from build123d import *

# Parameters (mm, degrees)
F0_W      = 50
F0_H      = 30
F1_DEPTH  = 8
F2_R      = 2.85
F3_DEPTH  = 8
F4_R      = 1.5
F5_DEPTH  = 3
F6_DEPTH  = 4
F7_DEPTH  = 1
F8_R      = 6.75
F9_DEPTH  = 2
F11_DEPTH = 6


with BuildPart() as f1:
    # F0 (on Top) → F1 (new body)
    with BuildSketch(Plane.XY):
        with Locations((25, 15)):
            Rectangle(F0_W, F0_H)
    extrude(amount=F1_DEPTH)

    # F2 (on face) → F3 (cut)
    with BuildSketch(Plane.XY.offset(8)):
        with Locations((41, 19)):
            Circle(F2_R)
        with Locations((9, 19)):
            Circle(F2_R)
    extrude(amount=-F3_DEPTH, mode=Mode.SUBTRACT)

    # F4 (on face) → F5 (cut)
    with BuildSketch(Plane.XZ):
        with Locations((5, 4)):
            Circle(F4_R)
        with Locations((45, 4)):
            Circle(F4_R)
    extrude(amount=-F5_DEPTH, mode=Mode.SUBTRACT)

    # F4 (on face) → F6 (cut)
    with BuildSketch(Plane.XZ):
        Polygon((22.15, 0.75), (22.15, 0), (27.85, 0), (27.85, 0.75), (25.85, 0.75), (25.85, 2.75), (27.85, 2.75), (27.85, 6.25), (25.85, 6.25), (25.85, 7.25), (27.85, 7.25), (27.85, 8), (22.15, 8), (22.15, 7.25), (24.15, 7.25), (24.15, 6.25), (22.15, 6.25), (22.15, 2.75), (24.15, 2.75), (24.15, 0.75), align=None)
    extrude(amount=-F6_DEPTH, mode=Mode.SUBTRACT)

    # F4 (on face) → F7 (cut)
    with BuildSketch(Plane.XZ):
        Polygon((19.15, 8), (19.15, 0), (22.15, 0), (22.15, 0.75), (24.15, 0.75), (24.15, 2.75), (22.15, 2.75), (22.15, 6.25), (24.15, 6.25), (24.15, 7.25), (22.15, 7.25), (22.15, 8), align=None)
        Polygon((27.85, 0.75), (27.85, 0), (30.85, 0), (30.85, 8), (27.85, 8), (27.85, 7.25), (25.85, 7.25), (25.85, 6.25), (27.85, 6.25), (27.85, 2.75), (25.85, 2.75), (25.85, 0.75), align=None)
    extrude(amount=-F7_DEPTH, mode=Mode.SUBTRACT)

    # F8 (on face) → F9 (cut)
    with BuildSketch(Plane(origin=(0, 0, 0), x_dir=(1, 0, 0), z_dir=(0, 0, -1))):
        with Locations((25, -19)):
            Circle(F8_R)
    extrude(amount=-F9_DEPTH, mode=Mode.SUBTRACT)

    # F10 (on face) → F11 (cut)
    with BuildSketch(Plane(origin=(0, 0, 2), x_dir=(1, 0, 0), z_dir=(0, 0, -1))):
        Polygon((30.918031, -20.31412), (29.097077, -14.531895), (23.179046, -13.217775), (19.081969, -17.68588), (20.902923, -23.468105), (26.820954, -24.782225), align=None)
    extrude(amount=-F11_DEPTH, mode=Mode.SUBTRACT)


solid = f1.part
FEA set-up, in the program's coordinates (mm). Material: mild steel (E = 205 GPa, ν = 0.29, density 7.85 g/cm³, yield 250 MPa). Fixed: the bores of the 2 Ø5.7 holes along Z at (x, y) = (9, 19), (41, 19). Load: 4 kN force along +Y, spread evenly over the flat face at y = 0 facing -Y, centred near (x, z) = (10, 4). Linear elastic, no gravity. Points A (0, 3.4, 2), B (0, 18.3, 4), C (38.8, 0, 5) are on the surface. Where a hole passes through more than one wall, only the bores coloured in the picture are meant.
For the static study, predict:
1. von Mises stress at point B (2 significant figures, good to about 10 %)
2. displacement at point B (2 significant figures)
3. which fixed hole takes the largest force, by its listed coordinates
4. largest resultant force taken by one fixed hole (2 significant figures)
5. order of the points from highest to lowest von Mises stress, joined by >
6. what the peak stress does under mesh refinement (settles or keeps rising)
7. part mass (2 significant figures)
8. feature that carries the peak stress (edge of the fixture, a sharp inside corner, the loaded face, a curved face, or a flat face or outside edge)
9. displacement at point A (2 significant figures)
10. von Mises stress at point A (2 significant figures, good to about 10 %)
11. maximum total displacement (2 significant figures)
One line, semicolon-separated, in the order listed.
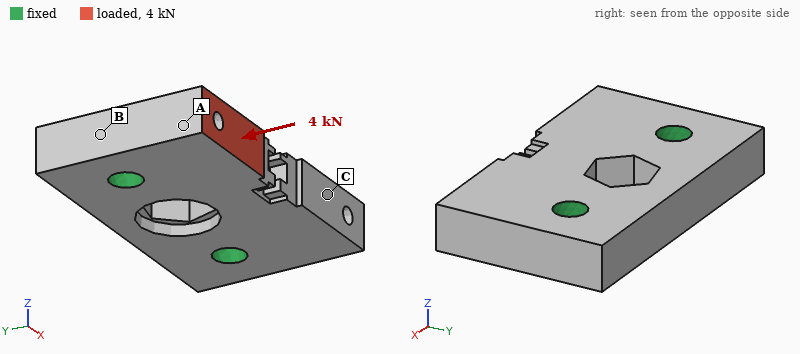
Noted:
15 MPa; 1.0 µm; (9, 19); 3.8 kN; A > B > C; keeps rising; 82 g; edge of the fixture; 2.7 µm; 27 MPa; 3.2 µm
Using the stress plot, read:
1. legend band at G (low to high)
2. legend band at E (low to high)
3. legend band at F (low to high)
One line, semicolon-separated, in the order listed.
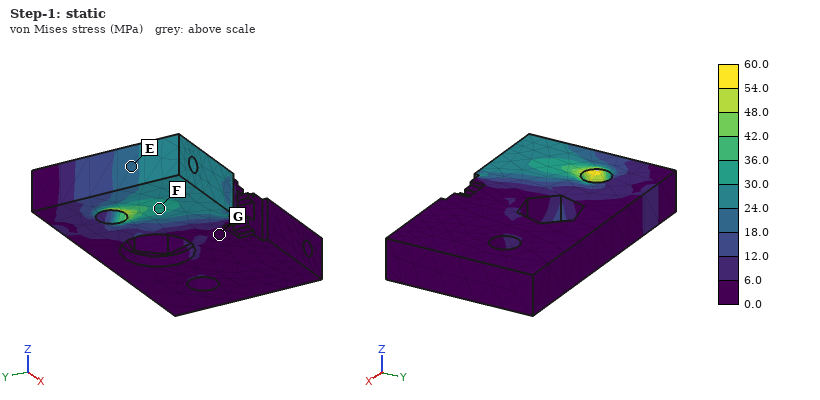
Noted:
0.0 to 6.0 MPa; 18.0 to 24.0 MPa; 30.0 to 36.0 MPa
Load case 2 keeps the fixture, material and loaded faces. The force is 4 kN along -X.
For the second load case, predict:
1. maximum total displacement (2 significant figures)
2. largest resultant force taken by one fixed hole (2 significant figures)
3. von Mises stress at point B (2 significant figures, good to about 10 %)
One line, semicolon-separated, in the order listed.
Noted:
13 µm; 2.8 kN; 35 MPa
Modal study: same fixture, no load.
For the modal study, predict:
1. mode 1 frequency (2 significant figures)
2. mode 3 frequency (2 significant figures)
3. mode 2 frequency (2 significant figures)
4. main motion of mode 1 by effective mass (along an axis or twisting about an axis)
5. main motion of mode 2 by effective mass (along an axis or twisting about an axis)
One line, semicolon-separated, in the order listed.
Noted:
15 kHz; 28 kHz; 21 kHz; along Z; twisting about Y
